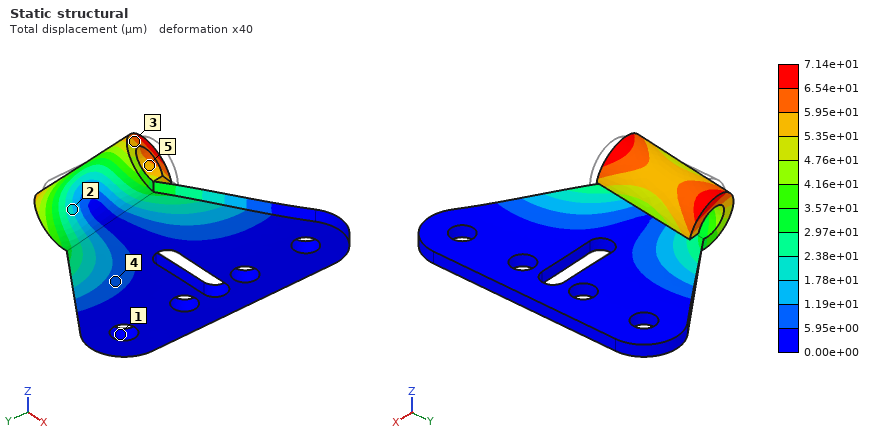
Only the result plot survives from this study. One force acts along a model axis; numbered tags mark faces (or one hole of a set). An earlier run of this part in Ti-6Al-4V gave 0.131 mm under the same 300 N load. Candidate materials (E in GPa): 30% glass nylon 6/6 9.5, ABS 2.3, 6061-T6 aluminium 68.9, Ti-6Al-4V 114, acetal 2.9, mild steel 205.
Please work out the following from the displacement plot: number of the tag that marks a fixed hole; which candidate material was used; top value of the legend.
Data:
1
mild steel
7.14e+01 µm
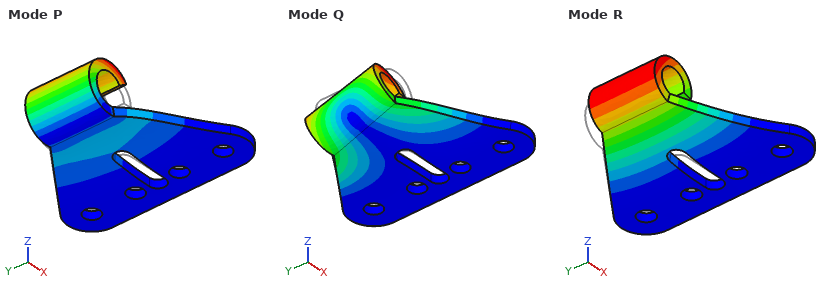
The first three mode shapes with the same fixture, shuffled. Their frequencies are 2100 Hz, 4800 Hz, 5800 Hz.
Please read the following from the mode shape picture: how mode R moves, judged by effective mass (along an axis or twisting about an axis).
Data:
along Z
